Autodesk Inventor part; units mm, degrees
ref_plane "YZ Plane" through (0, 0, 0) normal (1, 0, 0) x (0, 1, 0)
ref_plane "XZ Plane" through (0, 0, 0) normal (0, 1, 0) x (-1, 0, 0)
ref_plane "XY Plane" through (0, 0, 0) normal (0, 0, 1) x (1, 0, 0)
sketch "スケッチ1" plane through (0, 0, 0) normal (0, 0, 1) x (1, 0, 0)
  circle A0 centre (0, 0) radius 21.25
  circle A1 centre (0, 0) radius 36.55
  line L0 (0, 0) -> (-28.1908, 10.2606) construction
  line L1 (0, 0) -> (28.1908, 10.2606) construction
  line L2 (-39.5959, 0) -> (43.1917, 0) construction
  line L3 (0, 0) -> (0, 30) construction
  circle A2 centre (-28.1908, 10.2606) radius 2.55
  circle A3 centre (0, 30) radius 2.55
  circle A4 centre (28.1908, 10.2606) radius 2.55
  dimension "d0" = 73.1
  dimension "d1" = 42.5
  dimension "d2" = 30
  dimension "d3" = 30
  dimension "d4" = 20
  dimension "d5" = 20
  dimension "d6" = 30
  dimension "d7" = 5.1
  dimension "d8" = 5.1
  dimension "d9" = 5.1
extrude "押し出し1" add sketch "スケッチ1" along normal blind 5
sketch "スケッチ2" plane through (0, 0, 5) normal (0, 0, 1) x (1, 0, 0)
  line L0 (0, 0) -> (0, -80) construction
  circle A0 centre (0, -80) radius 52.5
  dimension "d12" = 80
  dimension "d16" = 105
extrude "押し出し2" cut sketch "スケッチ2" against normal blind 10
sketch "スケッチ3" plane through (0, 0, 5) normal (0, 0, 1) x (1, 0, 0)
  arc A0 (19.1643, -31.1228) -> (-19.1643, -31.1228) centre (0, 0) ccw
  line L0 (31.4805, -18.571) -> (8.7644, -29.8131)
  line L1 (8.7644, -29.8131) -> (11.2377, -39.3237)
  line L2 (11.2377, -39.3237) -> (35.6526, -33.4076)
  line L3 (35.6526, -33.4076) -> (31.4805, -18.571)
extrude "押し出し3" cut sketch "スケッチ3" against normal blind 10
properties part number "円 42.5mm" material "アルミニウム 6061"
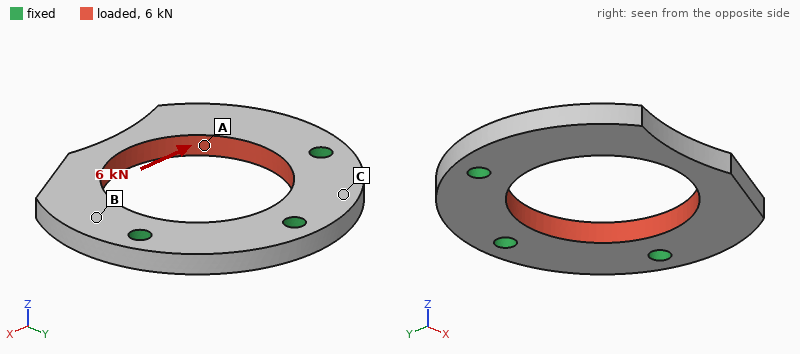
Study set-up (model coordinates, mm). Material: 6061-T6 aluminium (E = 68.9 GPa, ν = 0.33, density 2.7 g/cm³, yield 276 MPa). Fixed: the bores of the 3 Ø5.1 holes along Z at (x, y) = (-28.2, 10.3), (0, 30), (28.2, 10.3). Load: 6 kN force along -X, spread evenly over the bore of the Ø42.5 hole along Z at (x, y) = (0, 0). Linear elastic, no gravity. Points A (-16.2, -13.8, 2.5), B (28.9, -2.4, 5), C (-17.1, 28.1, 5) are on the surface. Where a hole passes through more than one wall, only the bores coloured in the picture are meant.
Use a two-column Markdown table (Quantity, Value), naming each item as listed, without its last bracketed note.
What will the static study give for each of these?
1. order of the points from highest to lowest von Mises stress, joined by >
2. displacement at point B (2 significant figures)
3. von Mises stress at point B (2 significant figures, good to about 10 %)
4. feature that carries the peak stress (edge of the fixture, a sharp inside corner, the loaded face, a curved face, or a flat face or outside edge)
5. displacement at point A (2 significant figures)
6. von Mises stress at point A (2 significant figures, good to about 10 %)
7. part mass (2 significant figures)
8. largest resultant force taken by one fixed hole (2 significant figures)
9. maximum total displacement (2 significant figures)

| Quantity | Value |
|---|---|
| order of the points from highest to lowest von Mises stress, joined by > | A > B > C |
| displacement at point B | 35 µm |
| von Mises stress at point B | 46 MPa |
| feature that carries the peak stress | edge of the fixture |
| displacement at point A | 76 µm |
| von Mises stress at point A | 80 MPa |
| part mass | 32 g |
| largest resultant force taken by one fixed hole | 2.8 kN |
| maximum total displacement | 98 µm |
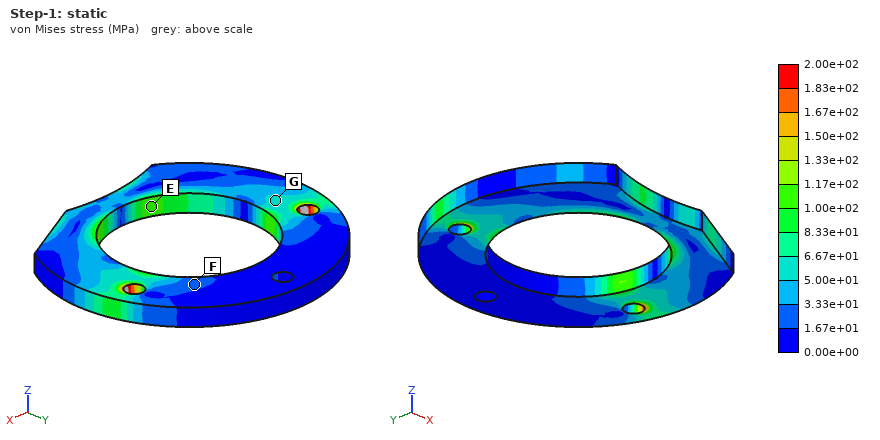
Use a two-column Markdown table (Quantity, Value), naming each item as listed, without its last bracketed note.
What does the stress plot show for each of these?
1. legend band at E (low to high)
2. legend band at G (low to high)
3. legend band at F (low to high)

| Quantity | Value |
|---|---|
| legend band at E | 1.00e+02 to 1.17e+02 MPa |
| legend band at G | 5.00e+01 to 6.67e+01 MPa |
| legend band at F | 1.67e+01 to 3.33e+01 MPa |
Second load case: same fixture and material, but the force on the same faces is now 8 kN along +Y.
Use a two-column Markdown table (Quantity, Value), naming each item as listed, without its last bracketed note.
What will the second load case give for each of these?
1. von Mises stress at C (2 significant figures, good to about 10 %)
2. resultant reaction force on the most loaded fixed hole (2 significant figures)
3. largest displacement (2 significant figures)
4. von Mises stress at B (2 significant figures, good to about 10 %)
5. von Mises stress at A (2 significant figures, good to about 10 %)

| Quantity | Value |
|---|---|
| von Mises stress at C | 8.6 MPa |
| resultant reaction force on the most loaded fixed hole | 3.3 kN |
| largest displacement | 51 µm |
| von Mises stress at B | 33 MPa |
| von Mises stress at A | 70 MPa |
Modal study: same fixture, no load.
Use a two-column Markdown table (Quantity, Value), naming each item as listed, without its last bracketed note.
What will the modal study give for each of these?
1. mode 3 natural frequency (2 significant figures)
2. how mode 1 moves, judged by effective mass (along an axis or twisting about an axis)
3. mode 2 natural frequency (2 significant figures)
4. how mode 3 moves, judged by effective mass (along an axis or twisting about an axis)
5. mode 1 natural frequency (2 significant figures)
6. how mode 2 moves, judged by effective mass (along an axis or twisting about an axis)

| Quantity | Value |
|---|---|
| mode 3 natural frequency | 8100 Hz |
| how mode 1 moves, judged by effective mass | along Z |
| mode 2 natural frequency | 4700 Hz |
| how mode 3 moves, judged by effective mass | along X |
| mode 1 natural frequency | 2300 Hz |
| how mode 2 moves, judged by effective mass | twisting about Y |
